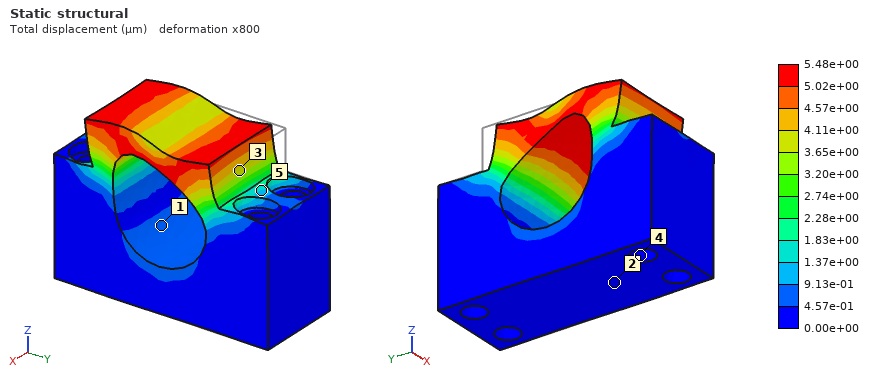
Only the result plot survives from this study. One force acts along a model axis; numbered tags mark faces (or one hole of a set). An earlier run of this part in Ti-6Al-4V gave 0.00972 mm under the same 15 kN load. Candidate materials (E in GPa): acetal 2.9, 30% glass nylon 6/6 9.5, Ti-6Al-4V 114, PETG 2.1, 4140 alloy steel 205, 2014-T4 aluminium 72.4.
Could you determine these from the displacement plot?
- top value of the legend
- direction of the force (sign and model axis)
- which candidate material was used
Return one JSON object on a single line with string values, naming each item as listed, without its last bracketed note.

{"top value of the legend": "5.48e+00 µm", "direction of the force": "-Y", "which candidate material was used": "4140 alloy steel"}
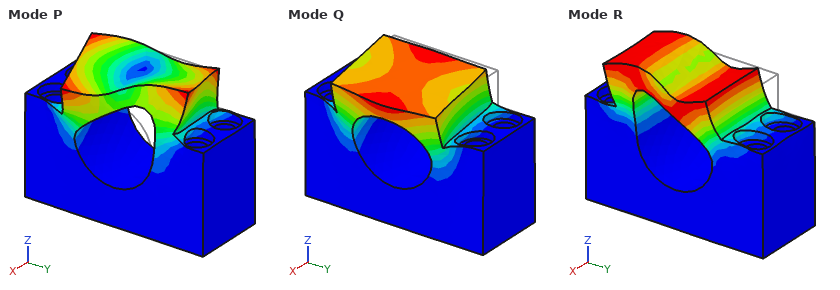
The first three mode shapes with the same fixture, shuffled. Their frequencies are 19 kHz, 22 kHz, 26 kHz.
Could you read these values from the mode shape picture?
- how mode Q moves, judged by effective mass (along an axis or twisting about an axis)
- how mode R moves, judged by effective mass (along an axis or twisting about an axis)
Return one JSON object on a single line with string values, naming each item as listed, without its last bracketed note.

{"how mode Q moves, judged by effective mass": "along X", "how mode R moves, judged by effective mass": "along Y"}
